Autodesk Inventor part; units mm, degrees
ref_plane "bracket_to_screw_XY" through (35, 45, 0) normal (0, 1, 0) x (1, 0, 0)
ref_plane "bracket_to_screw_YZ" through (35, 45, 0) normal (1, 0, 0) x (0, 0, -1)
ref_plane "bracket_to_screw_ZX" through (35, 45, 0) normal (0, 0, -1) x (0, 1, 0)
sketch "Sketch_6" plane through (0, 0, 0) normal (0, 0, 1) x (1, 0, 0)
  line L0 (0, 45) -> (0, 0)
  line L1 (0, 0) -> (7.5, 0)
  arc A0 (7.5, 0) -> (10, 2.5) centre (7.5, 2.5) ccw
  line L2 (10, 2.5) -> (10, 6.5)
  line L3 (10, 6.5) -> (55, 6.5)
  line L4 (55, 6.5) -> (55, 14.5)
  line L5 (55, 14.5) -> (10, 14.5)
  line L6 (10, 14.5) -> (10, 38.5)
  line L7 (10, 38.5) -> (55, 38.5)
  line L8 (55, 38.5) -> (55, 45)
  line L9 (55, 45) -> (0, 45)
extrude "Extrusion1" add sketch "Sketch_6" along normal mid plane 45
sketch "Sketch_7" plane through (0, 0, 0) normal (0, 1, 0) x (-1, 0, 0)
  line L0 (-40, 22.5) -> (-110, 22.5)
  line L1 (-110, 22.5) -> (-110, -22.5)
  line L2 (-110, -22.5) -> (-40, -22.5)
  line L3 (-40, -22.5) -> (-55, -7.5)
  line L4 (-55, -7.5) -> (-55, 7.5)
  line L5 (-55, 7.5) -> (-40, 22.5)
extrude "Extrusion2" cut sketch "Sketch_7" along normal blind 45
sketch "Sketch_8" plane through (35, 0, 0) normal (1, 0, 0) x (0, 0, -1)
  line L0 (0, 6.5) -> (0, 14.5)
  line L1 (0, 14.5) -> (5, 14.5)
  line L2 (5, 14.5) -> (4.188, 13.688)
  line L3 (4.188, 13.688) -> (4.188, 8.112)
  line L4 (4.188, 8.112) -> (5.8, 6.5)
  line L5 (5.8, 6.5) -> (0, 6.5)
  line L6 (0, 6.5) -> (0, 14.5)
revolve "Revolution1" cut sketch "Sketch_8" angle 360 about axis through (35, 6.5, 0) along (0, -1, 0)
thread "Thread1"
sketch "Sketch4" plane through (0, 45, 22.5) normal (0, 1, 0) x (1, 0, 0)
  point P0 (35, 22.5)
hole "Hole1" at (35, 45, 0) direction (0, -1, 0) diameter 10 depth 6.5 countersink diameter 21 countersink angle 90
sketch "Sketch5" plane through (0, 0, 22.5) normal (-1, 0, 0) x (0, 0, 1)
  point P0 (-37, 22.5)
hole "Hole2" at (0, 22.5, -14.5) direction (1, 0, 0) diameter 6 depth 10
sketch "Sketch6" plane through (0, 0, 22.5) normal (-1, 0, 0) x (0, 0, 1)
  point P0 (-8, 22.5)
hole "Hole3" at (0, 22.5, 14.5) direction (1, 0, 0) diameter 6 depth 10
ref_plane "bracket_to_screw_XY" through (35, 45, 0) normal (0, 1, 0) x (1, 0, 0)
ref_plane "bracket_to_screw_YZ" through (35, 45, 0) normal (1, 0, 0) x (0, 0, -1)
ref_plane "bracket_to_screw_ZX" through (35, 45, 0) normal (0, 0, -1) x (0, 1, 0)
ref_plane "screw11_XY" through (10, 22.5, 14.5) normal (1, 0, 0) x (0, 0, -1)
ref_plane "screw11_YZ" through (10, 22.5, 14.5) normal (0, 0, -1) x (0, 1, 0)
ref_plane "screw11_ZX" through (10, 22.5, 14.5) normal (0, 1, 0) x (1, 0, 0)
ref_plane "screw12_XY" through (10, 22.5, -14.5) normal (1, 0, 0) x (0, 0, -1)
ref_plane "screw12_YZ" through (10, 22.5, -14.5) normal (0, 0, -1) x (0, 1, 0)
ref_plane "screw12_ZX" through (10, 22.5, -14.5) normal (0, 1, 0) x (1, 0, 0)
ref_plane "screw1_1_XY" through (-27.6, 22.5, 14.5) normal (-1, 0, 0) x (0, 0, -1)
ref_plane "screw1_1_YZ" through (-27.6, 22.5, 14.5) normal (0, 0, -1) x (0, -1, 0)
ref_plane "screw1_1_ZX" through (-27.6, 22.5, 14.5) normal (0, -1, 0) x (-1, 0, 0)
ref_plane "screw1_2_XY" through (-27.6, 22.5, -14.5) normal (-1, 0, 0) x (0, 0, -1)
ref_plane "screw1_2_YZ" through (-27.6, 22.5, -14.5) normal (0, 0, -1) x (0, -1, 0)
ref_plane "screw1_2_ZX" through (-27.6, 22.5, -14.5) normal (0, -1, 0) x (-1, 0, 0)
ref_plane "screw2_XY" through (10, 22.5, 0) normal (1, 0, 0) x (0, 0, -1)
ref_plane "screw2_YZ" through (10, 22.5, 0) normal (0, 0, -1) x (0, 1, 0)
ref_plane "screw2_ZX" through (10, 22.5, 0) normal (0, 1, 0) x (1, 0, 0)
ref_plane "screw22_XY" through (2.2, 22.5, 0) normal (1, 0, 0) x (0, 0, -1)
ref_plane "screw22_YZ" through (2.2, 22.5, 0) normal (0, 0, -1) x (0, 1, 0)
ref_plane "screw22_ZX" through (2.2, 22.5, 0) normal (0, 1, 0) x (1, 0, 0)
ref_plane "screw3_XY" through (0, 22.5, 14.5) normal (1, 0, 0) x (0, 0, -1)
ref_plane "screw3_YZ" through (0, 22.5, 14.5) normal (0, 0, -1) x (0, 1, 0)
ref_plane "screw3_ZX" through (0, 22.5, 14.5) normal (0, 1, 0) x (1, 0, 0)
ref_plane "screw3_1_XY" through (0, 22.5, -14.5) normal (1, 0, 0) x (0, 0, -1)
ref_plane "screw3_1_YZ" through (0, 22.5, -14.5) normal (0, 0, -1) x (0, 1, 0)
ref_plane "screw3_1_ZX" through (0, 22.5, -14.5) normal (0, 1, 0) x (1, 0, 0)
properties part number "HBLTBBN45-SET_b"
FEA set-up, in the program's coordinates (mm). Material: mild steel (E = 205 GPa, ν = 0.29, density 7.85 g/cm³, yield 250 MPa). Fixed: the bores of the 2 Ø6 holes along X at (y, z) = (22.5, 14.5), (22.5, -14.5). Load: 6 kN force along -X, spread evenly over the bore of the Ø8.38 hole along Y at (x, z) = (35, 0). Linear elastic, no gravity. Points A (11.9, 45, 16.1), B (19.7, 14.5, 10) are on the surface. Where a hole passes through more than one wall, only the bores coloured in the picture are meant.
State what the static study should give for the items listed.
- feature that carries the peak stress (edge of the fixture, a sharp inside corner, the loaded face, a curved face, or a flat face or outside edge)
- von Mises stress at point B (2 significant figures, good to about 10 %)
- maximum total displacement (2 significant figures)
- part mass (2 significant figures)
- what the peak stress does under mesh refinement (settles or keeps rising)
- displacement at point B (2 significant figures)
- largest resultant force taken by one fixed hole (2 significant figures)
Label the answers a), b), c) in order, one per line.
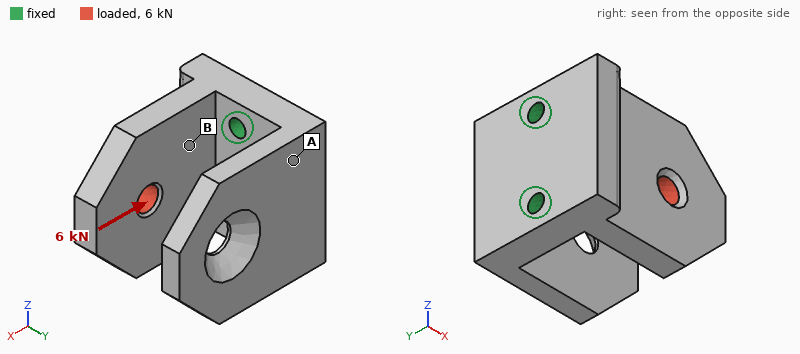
a) edge of the fixture
b) 24 MPa
c) 27 µm
d) 350 g
e) keeps rising
f) 9.9 µm
g) 3.0 kN
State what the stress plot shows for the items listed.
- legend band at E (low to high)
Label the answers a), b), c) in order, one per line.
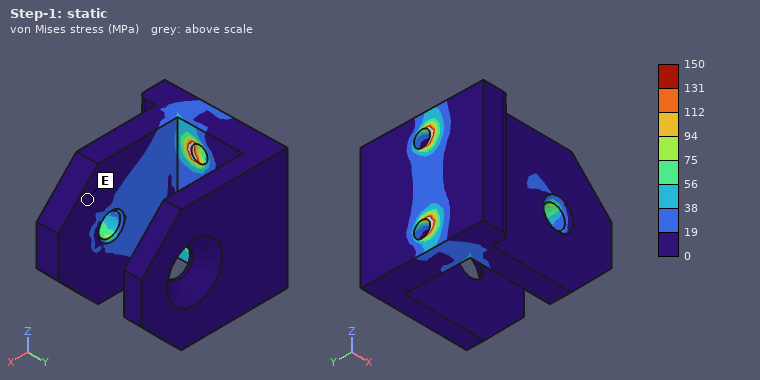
a) 0 to 19 MPa
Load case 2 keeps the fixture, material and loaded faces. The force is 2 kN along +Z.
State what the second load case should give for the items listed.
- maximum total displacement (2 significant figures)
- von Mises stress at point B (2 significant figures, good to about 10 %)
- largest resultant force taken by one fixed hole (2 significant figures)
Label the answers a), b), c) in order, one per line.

a) 14 µm
b) 18 MPa
c) 2.1 kN
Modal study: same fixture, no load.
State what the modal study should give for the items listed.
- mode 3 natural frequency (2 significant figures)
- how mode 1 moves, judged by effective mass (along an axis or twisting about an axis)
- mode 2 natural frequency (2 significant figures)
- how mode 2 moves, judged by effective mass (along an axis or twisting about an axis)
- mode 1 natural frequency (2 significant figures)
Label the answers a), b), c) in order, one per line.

a) 5300 Hz
b) along Y
c) 2800 Hz
d) along Y
e) 2400 Hz
